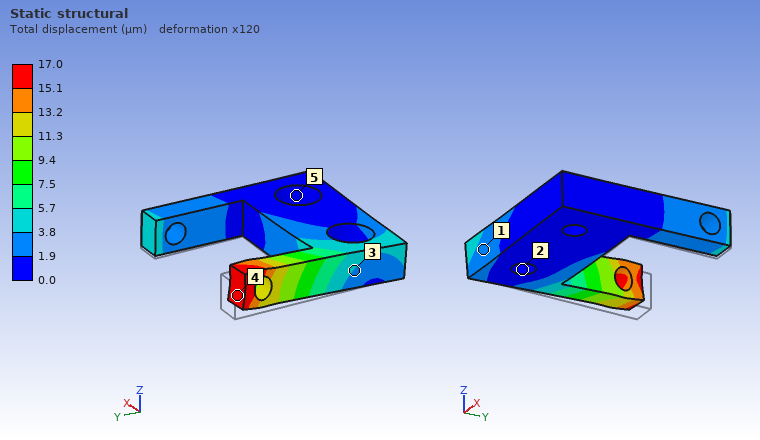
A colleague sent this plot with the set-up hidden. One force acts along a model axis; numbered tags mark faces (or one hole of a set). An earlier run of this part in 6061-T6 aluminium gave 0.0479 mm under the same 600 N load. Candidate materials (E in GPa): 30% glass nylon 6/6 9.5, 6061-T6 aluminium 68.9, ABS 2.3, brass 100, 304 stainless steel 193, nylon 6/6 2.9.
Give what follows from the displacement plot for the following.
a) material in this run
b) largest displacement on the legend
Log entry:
304 stainless steel
17.0 µm
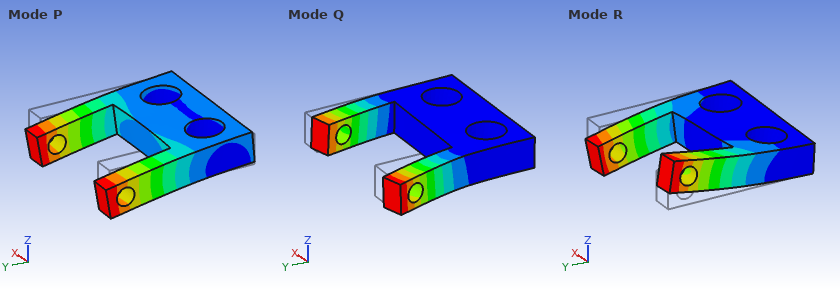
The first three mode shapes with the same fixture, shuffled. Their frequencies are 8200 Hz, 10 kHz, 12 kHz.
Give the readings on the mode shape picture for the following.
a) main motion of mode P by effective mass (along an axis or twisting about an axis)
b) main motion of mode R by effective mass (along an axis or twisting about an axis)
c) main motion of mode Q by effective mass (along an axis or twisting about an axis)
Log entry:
along Z
twisting about Y
along X
